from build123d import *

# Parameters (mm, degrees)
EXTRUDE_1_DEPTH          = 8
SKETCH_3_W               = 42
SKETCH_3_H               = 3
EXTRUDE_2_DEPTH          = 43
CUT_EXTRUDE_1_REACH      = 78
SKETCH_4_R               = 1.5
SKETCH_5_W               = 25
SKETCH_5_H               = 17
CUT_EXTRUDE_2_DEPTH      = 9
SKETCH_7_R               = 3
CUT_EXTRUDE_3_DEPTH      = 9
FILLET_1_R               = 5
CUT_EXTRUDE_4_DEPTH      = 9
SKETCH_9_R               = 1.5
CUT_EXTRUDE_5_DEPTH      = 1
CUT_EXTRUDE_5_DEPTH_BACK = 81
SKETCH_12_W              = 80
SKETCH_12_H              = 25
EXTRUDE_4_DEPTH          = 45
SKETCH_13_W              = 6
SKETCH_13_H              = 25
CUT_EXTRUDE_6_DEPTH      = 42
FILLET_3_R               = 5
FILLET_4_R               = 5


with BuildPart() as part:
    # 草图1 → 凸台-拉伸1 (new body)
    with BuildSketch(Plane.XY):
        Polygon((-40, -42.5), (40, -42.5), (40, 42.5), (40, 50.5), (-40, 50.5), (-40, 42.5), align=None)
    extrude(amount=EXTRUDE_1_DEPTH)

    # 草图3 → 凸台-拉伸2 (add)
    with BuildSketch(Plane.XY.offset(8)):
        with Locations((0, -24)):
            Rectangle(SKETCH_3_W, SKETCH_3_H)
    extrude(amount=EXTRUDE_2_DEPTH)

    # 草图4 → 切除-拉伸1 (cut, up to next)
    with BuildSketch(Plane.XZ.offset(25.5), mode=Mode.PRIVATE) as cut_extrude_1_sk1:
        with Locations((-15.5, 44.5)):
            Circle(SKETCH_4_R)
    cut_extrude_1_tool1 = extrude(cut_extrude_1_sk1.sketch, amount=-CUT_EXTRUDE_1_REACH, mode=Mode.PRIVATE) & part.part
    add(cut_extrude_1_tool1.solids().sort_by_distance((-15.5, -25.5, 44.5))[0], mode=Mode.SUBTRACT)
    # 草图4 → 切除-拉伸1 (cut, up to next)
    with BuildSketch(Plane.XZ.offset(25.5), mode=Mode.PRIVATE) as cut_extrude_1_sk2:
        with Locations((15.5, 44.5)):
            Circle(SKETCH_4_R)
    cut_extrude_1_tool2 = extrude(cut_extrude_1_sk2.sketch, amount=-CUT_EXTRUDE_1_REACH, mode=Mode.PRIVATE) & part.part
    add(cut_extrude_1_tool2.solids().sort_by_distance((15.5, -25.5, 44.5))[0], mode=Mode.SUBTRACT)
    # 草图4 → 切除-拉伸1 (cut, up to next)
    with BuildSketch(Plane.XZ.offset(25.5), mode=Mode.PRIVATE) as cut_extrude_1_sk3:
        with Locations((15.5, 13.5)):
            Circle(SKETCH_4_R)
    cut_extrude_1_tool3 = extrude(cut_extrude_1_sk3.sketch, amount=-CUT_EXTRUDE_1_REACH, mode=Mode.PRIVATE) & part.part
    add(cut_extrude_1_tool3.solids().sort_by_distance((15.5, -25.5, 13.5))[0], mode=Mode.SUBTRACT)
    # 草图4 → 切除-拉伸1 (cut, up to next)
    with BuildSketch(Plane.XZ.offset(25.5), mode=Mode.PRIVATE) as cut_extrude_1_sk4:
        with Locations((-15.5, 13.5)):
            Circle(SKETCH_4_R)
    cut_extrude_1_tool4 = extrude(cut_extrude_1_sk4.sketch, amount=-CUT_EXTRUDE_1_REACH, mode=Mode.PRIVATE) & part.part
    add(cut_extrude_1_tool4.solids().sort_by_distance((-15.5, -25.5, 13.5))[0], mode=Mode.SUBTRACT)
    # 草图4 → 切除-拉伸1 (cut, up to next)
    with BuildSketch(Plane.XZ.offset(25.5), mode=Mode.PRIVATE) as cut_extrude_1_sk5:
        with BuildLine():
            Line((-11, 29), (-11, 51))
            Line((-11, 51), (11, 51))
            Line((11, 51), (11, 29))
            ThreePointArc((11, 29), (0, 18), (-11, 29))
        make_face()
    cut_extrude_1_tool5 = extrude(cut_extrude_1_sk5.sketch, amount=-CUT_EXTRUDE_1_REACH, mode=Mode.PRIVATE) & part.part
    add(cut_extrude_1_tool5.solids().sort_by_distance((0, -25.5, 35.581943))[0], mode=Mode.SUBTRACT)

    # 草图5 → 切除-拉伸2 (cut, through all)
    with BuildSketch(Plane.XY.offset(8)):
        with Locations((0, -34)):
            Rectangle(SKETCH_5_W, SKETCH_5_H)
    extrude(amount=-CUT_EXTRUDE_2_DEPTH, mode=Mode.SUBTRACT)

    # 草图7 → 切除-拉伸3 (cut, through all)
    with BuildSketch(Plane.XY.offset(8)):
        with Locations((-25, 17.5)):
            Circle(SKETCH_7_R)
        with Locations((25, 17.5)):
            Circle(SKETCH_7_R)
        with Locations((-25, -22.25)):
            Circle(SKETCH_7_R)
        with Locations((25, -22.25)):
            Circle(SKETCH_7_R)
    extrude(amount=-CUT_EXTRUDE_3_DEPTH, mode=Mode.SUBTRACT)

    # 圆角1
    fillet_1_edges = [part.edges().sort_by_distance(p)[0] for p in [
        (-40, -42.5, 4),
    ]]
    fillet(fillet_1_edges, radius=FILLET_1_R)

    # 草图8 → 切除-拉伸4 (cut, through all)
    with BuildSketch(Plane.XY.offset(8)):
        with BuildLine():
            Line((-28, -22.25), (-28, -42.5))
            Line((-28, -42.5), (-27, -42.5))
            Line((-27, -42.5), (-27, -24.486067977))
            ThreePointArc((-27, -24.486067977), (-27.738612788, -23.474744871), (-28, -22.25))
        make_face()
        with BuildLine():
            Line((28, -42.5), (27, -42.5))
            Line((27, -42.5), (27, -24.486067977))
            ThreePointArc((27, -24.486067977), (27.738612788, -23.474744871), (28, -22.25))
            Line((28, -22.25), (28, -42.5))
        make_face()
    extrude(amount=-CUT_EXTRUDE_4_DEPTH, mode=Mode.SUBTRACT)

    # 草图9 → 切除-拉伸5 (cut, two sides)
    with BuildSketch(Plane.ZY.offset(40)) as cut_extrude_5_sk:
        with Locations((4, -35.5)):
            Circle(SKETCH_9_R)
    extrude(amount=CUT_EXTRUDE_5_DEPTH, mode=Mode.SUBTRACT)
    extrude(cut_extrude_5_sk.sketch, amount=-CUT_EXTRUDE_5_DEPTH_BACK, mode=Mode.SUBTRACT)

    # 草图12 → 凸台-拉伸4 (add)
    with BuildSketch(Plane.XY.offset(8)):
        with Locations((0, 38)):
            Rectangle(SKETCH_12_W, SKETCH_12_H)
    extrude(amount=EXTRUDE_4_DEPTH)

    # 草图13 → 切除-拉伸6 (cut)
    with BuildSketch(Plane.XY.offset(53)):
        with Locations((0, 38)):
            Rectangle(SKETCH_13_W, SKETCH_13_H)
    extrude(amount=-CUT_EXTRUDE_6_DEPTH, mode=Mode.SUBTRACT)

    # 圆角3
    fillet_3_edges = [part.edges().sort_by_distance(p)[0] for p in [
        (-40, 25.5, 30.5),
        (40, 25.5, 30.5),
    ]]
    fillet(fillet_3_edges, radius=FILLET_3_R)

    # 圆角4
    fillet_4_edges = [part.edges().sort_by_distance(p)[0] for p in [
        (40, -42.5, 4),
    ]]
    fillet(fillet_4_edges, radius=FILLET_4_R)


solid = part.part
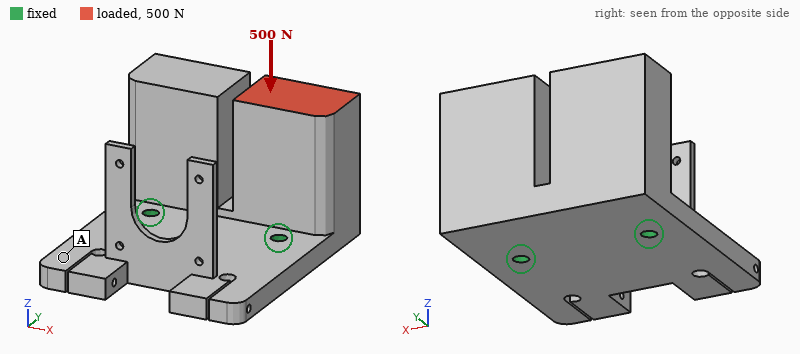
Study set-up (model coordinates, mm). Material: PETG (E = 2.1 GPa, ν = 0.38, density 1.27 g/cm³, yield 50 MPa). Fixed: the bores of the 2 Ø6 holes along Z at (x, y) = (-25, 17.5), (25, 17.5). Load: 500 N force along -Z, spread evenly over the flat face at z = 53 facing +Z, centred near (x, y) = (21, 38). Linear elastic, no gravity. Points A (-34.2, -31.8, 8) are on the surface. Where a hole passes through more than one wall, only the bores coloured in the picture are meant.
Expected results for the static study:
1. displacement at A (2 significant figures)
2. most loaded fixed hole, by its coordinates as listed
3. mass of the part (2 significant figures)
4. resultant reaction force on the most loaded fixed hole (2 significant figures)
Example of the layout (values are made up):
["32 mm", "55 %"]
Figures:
["0.19 mm", "(25, 17.5)", "180 g", "440 N"]
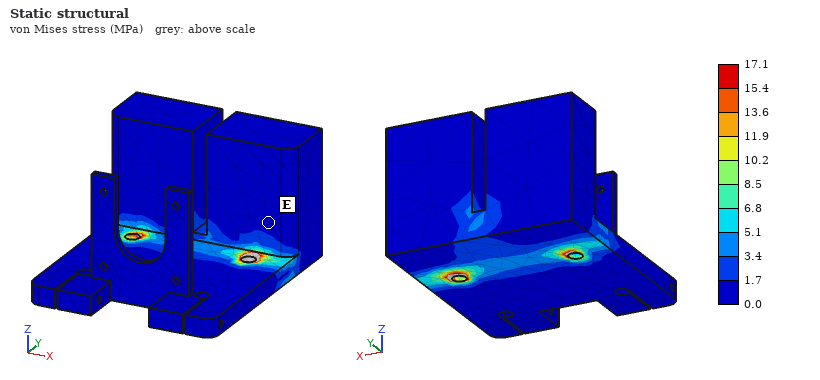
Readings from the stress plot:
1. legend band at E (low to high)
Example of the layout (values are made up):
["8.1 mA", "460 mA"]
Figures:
["0.0 to 1.7 MPa"]
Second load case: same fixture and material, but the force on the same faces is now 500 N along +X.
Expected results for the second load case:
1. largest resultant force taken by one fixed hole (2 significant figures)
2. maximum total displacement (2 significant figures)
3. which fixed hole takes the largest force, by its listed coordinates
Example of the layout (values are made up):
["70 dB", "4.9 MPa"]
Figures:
["570 N", "0.87 mm", "(-25, 17.5)"]
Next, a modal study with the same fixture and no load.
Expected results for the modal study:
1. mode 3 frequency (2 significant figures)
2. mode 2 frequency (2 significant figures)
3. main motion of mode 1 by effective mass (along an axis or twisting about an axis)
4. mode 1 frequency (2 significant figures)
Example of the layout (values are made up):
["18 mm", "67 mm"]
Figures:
["410 Hz", "370 Hz", "along Y", "310 Hz"]
